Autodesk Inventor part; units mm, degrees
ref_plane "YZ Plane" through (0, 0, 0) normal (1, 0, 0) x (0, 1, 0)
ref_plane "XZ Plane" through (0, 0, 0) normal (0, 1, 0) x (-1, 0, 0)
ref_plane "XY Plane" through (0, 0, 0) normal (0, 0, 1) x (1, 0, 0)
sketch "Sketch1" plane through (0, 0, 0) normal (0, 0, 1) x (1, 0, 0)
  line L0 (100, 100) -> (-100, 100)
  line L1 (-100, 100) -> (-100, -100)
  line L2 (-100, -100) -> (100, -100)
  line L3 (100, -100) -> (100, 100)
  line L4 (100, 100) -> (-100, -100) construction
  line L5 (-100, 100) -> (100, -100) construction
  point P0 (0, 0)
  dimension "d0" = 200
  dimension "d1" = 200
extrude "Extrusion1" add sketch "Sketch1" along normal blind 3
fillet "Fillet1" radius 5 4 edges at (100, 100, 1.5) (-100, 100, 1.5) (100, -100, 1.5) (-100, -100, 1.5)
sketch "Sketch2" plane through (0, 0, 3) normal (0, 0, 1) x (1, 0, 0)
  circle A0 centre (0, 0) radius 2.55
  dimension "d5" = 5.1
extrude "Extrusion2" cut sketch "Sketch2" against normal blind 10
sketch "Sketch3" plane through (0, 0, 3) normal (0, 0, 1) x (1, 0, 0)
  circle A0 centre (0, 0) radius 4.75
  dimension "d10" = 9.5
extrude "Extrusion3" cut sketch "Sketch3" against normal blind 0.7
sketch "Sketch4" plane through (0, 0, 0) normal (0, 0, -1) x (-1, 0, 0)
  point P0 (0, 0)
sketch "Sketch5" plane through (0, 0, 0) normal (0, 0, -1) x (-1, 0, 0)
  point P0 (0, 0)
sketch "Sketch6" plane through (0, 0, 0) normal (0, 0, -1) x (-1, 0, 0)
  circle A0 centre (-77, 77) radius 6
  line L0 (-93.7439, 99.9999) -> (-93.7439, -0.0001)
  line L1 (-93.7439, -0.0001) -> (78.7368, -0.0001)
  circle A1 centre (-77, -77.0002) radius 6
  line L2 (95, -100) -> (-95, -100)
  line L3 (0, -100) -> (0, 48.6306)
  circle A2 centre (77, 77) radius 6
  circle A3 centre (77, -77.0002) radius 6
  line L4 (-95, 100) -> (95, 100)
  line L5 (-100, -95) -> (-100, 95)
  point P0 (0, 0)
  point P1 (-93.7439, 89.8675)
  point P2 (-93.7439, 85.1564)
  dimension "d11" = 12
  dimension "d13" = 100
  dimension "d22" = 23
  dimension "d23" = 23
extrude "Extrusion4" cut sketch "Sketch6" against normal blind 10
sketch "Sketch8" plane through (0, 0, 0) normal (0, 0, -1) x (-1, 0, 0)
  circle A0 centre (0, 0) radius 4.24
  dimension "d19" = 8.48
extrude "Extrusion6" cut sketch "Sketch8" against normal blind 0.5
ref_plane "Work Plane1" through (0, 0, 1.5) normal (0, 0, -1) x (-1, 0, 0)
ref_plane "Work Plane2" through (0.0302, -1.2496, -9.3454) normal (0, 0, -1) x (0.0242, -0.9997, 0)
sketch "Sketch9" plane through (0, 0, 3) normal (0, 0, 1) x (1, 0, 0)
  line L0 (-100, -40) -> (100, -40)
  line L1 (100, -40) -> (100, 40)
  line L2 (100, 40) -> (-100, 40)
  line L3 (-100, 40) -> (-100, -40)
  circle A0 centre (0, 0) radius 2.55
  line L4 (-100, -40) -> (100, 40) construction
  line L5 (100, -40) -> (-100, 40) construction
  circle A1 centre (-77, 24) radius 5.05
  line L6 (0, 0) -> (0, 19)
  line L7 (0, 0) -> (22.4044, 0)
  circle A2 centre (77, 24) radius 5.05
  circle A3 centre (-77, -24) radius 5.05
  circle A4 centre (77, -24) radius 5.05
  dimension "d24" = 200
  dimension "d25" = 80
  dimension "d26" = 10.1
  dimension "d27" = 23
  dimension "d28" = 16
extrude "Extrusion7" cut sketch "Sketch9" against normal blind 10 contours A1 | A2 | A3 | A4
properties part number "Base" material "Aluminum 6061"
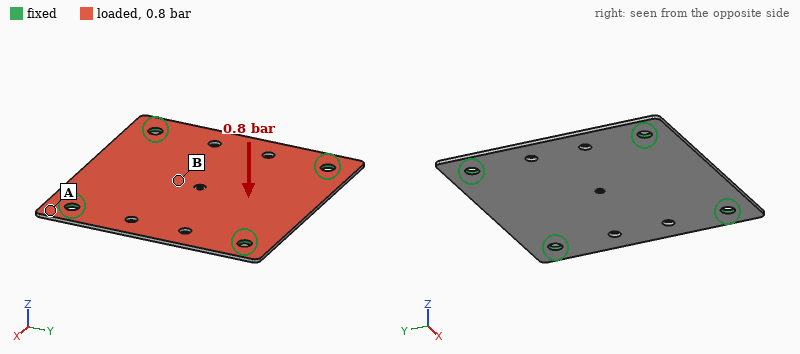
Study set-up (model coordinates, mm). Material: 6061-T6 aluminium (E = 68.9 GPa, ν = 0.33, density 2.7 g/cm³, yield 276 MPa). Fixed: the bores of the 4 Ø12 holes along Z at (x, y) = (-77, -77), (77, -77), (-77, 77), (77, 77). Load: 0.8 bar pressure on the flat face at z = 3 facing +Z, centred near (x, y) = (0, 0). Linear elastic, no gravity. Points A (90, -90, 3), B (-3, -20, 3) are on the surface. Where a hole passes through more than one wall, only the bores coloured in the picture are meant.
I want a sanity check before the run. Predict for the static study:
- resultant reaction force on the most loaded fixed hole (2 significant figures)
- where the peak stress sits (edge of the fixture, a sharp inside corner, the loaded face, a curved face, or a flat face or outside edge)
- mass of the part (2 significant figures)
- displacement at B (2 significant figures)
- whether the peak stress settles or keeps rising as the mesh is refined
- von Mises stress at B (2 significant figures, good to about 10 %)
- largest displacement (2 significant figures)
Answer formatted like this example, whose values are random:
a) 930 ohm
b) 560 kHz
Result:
a) 780 N
b) edge of the fixture
c) 320 g
d) 1.5 mm
e) keeps rising
f) 57 MPa
g) 1.6 mm
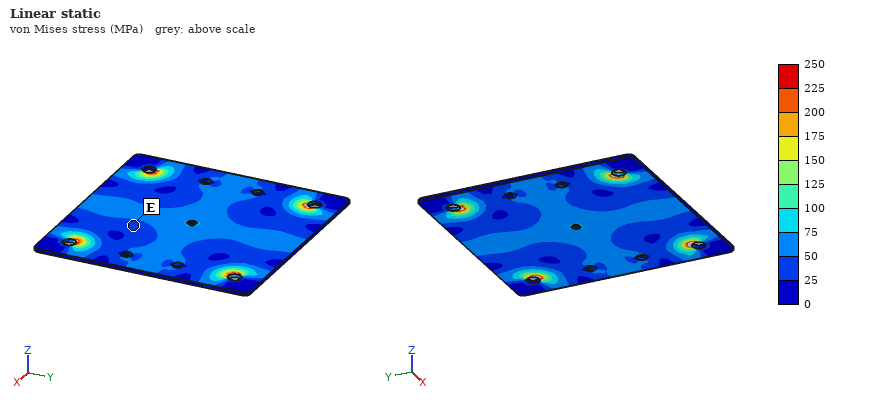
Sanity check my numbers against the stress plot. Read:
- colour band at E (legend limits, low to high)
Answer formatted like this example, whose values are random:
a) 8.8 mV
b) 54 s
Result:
a) 25 to 50 MPa
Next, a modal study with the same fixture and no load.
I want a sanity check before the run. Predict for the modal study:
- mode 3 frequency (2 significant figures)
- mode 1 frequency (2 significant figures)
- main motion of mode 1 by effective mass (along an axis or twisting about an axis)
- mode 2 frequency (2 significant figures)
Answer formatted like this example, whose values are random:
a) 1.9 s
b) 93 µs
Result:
a) 780 Hz
b) 490 Hz
c) along Z
d) 780 Hz
